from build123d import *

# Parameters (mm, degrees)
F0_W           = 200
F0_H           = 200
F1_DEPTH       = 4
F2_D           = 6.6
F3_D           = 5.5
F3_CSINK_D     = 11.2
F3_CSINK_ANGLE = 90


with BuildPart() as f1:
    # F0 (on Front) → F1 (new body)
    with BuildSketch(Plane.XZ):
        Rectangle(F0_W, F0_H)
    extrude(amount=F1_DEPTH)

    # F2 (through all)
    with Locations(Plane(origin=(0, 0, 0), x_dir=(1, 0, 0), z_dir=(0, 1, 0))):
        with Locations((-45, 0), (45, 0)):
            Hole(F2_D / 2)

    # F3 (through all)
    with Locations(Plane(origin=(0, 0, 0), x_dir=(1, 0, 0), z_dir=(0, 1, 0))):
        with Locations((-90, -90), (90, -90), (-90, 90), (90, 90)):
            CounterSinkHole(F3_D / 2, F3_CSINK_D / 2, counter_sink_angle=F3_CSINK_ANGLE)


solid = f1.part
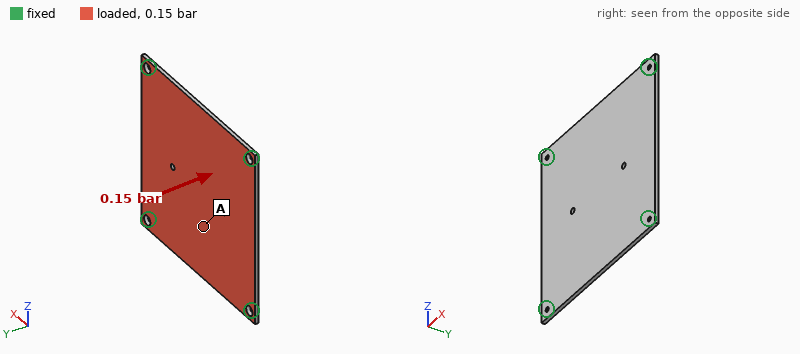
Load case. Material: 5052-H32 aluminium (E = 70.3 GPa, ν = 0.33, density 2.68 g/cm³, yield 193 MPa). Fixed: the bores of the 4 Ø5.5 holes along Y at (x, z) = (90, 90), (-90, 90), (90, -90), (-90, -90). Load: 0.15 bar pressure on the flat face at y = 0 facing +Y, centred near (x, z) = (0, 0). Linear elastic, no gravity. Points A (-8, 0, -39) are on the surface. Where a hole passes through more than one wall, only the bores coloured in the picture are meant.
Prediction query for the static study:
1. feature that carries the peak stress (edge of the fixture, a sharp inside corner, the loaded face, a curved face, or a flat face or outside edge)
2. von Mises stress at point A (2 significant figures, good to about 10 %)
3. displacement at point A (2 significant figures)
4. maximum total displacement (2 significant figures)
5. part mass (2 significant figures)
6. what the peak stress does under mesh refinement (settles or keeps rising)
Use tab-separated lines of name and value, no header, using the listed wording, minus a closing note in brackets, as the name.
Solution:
feature that carries the peak stress	edge of the fixture
von Mises stress at point A	12 MPa
displacement at point A	0.37 mm
maximum total displacement	0.42 mm
part mass	430 g
what the peak stress does under mesh refinement	keeps rising
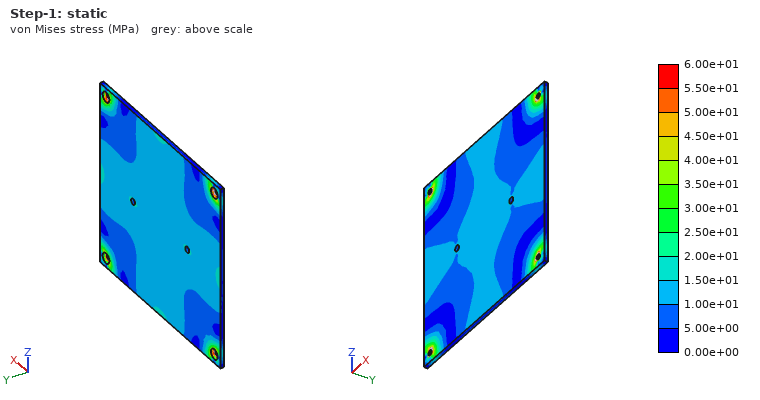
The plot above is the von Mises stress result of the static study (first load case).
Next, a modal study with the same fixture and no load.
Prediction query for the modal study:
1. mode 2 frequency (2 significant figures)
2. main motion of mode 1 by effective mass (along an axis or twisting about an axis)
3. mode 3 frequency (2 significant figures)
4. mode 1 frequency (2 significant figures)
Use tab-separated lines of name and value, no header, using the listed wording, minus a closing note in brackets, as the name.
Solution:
mode 2 frequency	630 Hz
main motion of mode 1 by effective mass	along Y
mode 3 frequency	630 Hz
mode 1 frequency	350 Hz
